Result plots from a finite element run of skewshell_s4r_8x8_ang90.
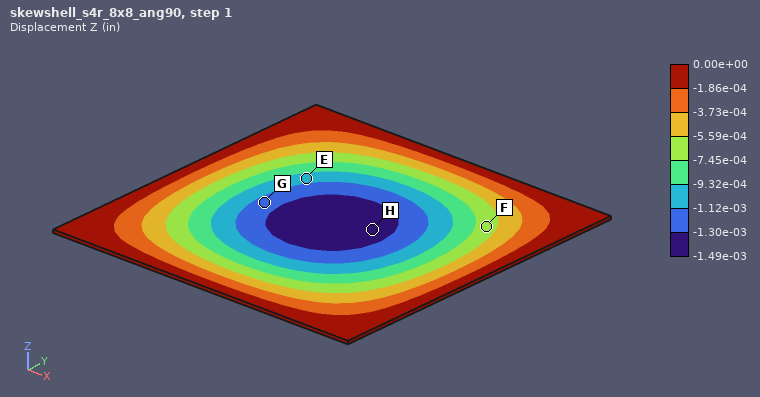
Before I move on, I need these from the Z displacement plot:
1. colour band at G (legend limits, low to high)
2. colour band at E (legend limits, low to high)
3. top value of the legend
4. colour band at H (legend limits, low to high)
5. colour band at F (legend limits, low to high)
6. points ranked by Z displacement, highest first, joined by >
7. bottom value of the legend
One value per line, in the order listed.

-1.30e-03 to -1.12e-03 in
-1.12e-03 to -9.32e-04 in
0.00e+00 in
-1.49e-03 to -1.30e-03 in
-7.45e-04 to -5.59e-04 in
F > E > G > H
-1.49e-03 in
